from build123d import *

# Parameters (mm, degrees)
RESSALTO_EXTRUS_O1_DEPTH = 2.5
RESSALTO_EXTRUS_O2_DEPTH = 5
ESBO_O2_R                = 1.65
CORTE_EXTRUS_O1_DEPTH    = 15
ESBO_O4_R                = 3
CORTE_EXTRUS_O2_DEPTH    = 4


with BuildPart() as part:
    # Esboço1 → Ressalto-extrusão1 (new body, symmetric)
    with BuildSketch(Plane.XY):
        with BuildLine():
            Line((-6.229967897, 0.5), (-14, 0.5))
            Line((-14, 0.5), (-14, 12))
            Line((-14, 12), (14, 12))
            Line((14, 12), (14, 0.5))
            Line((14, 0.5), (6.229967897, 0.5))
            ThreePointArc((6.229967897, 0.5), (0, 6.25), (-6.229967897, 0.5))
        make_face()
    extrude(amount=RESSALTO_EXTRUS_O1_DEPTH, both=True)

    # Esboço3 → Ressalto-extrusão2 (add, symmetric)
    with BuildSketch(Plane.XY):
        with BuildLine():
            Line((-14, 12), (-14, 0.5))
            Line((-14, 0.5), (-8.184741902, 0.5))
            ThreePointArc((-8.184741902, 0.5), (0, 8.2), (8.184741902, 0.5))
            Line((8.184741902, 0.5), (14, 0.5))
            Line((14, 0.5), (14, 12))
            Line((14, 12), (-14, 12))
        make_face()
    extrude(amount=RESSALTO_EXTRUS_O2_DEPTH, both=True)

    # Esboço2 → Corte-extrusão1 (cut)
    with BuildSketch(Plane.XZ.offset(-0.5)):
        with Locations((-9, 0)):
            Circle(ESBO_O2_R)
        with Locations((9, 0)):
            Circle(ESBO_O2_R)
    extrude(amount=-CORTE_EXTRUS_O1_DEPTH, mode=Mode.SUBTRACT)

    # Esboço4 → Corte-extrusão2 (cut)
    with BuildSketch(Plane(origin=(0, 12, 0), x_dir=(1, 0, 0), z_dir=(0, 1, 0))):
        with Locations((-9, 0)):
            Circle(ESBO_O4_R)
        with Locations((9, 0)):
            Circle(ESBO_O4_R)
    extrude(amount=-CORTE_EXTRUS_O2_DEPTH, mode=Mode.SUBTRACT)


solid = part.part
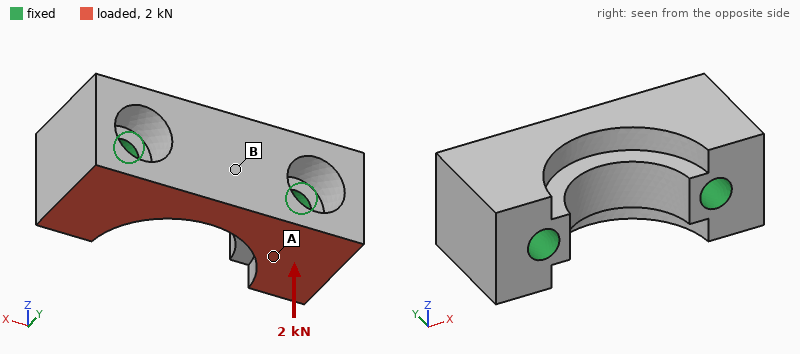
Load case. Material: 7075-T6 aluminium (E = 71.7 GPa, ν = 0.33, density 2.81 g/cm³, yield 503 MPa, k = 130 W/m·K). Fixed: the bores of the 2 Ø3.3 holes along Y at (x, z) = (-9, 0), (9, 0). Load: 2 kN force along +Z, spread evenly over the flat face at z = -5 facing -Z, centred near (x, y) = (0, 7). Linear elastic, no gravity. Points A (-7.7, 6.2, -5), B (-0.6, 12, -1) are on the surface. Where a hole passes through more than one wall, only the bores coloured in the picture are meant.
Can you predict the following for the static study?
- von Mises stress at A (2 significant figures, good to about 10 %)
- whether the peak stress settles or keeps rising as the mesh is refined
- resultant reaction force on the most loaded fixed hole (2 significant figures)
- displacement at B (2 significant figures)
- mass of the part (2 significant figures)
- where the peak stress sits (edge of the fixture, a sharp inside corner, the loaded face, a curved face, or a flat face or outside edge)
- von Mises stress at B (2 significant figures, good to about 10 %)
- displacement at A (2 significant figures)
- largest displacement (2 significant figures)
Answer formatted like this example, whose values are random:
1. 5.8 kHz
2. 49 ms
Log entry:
1. 31 MPa
2. keeps rising
3. 1.0 kN
4. 5.2 µm
5. 5.9 g
6. edge of the fixture
7. 6.5 MPa
8. 2.0 µm
9. 6.5 µm
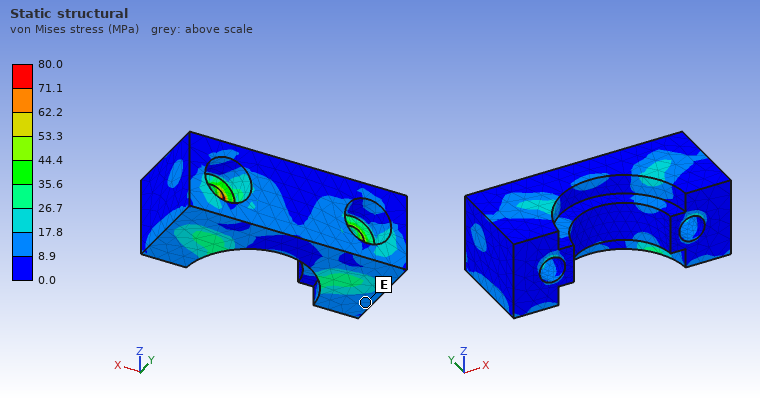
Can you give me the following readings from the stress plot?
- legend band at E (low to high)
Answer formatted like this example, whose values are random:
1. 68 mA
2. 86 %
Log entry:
1. 8.9 to 17.8 MPa
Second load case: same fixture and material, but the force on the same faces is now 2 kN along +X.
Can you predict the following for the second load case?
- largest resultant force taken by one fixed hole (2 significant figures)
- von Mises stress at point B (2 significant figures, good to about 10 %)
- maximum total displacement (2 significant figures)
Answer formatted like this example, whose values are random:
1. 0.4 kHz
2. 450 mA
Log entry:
1. 1.1 kN
2. 8.2 MPa
3. 6.7 µm
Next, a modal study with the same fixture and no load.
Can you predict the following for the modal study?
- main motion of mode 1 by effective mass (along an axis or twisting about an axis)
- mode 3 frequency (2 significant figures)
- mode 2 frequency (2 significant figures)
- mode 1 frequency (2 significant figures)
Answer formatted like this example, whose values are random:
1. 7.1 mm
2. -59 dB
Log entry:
1. along Z
2. 68 kHz
3. 66 kHz
4. 45 kHz
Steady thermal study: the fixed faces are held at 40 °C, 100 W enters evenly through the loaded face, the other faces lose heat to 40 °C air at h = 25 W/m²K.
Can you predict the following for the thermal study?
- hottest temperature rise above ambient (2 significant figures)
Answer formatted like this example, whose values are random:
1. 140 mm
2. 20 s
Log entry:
1. 31 K
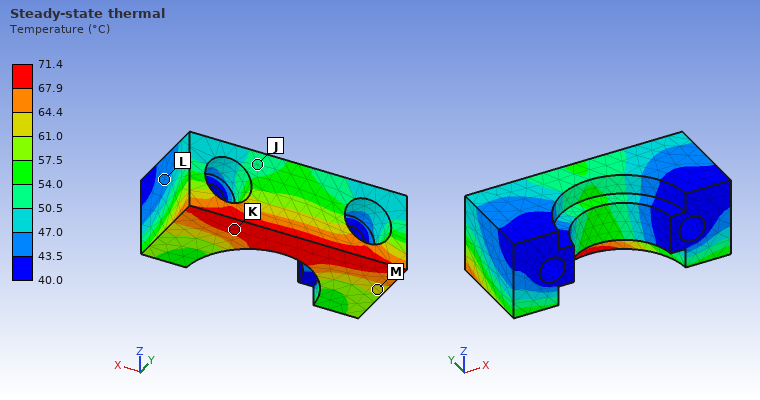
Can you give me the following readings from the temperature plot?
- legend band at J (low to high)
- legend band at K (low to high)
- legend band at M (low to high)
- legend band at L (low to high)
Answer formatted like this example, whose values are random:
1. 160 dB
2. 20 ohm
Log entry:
1. 50.5 to 54.0 °C
2. 67.9 to 71.4 °C
3. 61.0 to 64.4 °C
4. 43.5 to 47.0 °C
